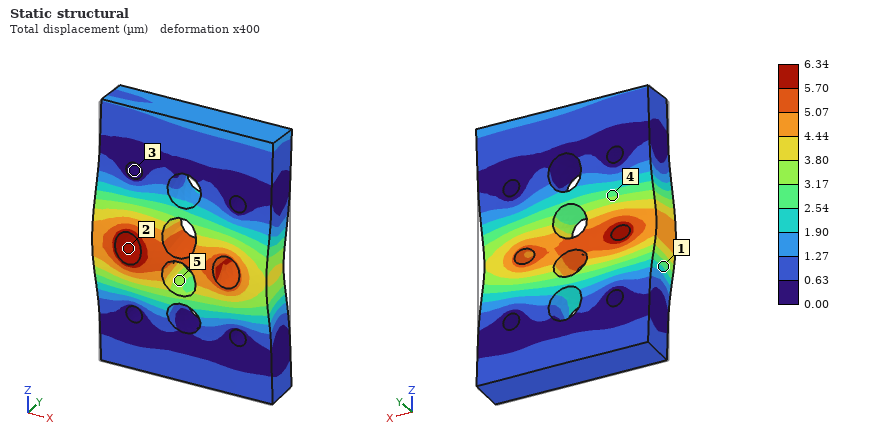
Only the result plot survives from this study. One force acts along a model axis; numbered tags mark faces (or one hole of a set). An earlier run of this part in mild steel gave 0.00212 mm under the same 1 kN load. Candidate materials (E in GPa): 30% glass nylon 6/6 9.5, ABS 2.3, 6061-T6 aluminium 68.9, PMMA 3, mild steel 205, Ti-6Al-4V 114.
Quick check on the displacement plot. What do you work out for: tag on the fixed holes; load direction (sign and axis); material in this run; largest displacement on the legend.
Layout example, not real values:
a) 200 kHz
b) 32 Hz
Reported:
a) 3
b) -Y
c) 6061-T6 aluminium
d) 6.34 µm
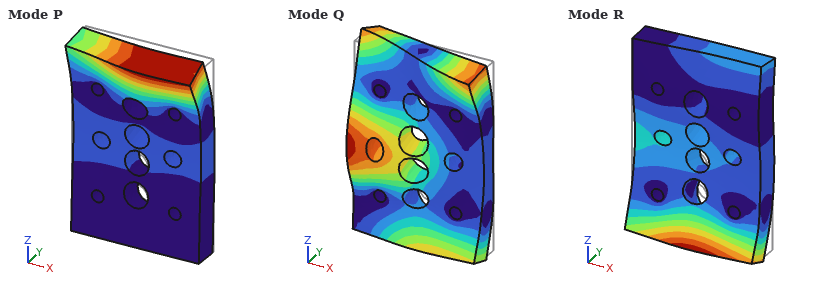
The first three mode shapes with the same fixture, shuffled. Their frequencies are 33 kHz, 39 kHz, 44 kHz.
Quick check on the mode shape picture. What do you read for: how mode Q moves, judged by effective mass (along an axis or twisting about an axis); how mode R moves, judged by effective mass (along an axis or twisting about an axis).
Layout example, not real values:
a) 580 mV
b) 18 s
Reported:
a) along Y
b) twisting about X
